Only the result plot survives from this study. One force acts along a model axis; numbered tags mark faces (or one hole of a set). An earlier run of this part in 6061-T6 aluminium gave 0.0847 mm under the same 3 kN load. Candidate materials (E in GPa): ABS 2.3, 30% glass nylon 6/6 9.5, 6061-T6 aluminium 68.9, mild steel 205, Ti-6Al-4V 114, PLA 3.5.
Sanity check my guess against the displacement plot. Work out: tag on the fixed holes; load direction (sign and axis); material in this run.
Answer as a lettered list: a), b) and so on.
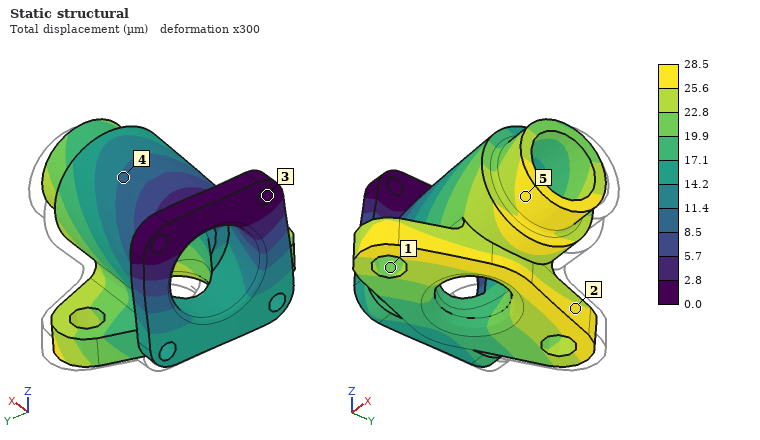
a) 3
b) -Y
c) mild steel
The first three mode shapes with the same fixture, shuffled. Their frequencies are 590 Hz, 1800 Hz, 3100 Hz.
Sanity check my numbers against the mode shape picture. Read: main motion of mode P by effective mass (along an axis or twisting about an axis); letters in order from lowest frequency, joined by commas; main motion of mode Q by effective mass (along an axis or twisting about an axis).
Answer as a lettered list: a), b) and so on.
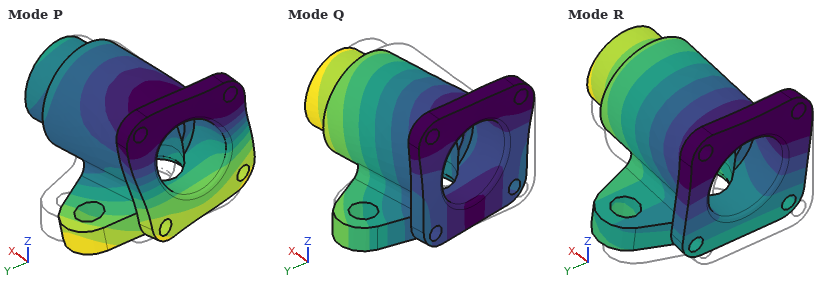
a) along Y
b) R, Q, P
c) along Y
